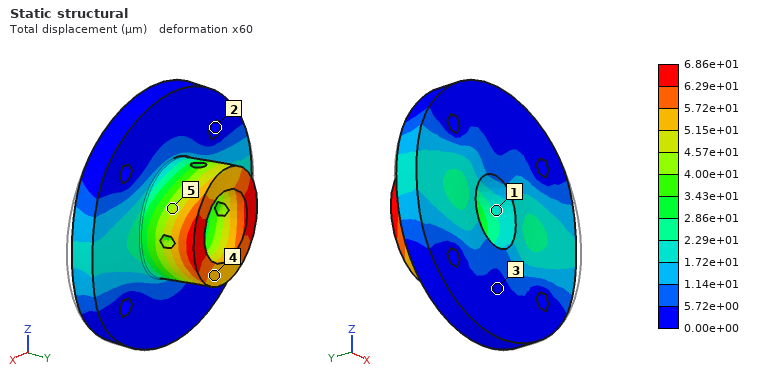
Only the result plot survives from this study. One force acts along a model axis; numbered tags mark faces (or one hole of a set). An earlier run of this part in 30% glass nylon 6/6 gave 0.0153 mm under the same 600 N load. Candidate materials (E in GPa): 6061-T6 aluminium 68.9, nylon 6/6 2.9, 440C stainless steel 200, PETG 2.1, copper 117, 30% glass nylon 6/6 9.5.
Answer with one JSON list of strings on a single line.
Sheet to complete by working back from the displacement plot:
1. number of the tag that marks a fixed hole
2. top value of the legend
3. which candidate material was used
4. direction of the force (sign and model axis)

["2", "6.86e+01 µm", "PETG", "-X"]
